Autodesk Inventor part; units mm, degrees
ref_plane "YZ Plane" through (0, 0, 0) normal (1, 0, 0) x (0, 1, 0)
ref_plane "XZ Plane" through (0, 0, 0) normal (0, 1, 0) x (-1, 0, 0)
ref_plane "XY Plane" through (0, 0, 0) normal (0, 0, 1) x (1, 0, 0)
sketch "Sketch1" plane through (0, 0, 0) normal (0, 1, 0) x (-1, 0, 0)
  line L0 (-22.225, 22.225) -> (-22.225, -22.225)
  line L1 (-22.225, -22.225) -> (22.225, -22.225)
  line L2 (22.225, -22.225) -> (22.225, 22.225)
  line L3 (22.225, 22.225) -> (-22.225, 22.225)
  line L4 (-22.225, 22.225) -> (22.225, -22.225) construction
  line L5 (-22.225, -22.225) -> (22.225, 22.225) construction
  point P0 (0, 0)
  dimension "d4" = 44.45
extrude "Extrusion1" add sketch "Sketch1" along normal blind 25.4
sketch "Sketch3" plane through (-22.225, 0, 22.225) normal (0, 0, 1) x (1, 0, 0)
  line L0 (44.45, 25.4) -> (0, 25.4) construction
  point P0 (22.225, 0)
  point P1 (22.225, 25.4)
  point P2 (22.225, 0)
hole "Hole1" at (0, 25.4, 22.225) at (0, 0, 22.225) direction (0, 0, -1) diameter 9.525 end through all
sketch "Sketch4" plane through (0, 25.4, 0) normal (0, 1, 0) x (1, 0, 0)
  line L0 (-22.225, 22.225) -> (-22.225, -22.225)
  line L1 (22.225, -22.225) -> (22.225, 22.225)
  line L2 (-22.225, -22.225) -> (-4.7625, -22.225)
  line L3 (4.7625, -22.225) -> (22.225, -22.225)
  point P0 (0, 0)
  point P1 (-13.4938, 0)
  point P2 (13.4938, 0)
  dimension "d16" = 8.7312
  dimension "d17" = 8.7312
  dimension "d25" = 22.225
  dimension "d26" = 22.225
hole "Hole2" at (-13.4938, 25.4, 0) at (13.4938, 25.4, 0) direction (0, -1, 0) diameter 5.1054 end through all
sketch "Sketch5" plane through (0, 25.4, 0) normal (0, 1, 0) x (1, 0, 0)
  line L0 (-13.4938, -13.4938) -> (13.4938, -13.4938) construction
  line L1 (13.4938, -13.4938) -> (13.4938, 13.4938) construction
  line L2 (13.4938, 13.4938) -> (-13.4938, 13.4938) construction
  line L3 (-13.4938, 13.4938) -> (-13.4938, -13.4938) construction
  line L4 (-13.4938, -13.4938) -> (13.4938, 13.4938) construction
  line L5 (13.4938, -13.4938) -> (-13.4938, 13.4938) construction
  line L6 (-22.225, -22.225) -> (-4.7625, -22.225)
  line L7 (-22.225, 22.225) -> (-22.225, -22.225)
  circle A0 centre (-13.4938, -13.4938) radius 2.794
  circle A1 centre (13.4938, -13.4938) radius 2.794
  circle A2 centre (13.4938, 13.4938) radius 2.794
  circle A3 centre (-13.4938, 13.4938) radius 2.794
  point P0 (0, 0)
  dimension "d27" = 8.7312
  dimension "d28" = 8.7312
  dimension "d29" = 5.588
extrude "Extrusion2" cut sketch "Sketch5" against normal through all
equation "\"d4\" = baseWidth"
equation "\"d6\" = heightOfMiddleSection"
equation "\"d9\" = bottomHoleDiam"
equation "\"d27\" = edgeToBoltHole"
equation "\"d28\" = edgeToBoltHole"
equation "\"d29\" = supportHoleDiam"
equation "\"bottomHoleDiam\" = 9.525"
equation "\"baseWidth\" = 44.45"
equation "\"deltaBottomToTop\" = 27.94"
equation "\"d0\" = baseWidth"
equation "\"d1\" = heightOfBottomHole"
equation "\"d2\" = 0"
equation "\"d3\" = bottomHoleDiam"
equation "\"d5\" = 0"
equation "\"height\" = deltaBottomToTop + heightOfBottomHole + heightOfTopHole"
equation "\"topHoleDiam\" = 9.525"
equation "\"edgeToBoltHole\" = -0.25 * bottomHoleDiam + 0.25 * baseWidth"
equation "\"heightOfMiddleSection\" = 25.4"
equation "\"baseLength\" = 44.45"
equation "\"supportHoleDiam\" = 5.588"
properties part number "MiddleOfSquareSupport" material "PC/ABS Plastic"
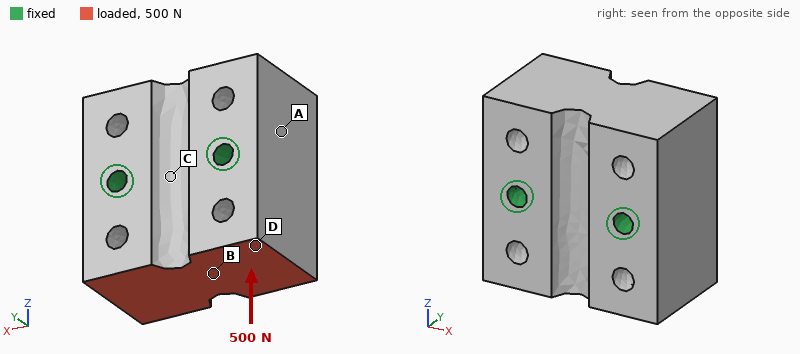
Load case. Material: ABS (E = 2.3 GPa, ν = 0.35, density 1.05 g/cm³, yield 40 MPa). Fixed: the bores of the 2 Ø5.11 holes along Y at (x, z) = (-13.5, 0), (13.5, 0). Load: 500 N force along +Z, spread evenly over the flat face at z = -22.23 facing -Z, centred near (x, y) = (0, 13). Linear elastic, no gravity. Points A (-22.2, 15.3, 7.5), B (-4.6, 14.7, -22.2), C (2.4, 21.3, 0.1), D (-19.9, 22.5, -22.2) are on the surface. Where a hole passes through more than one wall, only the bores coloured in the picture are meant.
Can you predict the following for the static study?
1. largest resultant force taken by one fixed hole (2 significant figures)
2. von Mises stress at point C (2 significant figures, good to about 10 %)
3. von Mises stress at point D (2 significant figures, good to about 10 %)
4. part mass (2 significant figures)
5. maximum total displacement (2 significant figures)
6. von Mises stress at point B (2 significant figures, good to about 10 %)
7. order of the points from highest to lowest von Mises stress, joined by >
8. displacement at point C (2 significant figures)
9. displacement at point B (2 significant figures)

250 N
0.23 MPa
0.46 MPa
46 g
6.9 µm
0.58 MPa
B > D > C > A
2.0 µm
5.5 µm
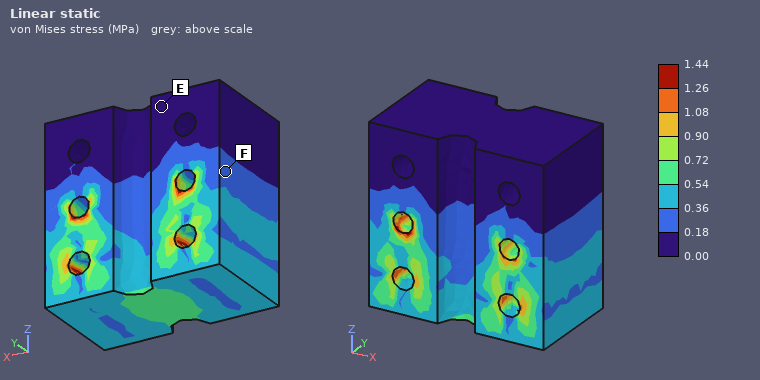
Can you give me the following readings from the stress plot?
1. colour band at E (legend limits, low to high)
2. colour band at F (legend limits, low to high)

0.00 to 0.18 MPa
0.18 to 0.36 MPa
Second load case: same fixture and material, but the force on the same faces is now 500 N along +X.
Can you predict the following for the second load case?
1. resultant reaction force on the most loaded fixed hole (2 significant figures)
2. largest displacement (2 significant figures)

430 N
32 µm
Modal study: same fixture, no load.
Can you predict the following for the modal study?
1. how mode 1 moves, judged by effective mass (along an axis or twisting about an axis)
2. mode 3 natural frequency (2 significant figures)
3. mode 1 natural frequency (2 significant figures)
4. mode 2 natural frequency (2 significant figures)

twisting about X
7200 Hz
6300 Hz
7100 Hz
